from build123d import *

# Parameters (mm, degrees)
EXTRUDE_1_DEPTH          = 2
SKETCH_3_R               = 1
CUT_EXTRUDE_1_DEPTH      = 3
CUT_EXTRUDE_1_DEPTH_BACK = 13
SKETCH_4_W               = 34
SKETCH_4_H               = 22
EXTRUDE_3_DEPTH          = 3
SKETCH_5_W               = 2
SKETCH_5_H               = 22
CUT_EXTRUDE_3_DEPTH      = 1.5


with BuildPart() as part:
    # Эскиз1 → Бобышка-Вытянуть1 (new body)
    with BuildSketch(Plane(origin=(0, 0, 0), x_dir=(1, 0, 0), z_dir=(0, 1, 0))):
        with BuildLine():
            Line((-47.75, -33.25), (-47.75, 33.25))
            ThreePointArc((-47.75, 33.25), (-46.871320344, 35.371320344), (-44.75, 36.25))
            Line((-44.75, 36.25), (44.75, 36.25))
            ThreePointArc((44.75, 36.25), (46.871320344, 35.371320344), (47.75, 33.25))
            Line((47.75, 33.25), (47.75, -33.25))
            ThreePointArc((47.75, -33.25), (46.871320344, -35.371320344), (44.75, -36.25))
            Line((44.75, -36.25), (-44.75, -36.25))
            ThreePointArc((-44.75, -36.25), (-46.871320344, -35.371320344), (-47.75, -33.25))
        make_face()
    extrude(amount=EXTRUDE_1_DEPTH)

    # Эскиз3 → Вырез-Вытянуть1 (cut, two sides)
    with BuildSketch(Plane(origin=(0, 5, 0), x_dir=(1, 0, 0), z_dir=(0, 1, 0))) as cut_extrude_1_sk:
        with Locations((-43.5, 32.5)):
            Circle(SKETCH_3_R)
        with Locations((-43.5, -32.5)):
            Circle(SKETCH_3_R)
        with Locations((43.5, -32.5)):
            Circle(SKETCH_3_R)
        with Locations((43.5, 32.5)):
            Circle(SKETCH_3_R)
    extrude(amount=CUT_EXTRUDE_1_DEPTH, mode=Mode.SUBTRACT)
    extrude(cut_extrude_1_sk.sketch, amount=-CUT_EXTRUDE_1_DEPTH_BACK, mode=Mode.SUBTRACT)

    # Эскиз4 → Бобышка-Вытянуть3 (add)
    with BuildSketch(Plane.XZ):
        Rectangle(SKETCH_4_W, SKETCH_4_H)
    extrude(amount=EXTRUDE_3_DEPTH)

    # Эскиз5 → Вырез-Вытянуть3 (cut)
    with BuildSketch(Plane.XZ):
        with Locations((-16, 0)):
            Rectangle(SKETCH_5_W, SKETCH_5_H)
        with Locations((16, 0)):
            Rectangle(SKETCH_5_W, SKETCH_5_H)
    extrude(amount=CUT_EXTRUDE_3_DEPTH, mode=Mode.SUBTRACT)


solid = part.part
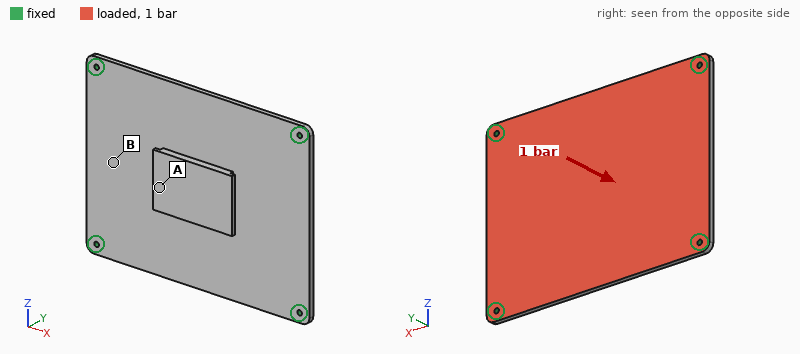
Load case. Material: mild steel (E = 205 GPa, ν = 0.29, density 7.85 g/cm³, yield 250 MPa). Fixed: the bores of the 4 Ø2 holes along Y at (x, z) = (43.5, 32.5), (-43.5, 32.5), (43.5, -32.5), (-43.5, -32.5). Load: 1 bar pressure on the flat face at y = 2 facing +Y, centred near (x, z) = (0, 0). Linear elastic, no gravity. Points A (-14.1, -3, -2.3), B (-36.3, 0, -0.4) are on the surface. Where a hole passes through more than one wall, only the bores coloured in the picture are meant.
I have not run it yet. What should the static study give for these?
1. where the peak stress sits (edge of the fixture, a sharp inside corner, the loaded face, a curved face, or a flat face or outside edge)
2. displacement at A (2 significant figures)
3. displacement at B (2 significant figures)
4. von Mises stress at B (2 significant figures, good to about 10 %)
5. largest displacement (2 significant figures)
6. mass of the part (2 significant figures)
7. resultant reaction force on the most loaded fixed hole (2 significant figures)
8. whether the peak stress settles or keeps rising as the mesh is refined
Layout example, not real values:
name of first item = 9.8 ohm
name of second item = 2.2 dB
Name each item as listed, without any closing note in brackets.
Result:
where the peak stress sits = edge of the fixture
displacement at A = 0.16 mm
displacement at B = 0.095 mm
von Mises stress at B = 41 MPa
largest displacement = 0.16 mm
mass of the part = 120 g
resultant reaction force on the most loaded fixed hole = 180 N
whether the peak stress settles or keeps rising as the mesh is refined = keeps rising
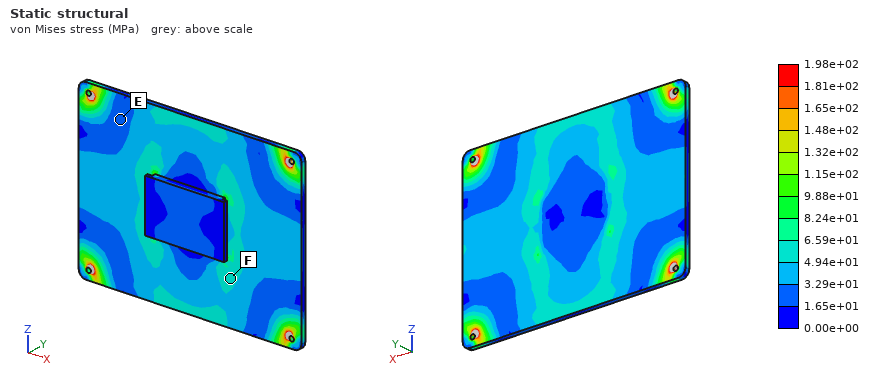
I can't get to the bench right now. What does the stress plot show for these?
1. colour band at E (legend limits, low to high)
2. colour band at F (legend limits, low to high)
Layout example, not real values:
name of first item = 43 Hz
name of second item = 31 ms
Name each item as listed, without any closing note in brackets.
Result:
colour band at E = 1.65e+01 to 3.29e+01 MPa
colour band at F = 4.94e+01 to 6.59e+01 MPa
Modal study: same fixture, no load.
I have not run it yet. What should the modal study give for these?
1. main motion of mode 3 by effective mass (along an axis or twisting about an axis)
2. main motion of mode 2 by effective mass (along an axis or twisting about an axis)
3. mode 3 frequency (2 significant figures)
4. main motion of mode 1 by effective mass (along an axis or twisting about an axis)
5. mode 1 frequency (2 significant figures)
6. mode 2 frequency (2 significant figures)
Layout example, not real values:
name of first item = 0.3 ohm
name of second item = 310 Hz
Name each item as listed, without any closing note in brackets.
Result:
main motion of mode 3 by effective mass = twisting about Z
main motion of mode 2 by effective mass = twisting about X
mode 3 frequency = 2200 Hz
main motion of mode 1 by effective mass = along Y
mode 1 frequency = 980 Hz
mode 2 frequency = 1700 Hz
